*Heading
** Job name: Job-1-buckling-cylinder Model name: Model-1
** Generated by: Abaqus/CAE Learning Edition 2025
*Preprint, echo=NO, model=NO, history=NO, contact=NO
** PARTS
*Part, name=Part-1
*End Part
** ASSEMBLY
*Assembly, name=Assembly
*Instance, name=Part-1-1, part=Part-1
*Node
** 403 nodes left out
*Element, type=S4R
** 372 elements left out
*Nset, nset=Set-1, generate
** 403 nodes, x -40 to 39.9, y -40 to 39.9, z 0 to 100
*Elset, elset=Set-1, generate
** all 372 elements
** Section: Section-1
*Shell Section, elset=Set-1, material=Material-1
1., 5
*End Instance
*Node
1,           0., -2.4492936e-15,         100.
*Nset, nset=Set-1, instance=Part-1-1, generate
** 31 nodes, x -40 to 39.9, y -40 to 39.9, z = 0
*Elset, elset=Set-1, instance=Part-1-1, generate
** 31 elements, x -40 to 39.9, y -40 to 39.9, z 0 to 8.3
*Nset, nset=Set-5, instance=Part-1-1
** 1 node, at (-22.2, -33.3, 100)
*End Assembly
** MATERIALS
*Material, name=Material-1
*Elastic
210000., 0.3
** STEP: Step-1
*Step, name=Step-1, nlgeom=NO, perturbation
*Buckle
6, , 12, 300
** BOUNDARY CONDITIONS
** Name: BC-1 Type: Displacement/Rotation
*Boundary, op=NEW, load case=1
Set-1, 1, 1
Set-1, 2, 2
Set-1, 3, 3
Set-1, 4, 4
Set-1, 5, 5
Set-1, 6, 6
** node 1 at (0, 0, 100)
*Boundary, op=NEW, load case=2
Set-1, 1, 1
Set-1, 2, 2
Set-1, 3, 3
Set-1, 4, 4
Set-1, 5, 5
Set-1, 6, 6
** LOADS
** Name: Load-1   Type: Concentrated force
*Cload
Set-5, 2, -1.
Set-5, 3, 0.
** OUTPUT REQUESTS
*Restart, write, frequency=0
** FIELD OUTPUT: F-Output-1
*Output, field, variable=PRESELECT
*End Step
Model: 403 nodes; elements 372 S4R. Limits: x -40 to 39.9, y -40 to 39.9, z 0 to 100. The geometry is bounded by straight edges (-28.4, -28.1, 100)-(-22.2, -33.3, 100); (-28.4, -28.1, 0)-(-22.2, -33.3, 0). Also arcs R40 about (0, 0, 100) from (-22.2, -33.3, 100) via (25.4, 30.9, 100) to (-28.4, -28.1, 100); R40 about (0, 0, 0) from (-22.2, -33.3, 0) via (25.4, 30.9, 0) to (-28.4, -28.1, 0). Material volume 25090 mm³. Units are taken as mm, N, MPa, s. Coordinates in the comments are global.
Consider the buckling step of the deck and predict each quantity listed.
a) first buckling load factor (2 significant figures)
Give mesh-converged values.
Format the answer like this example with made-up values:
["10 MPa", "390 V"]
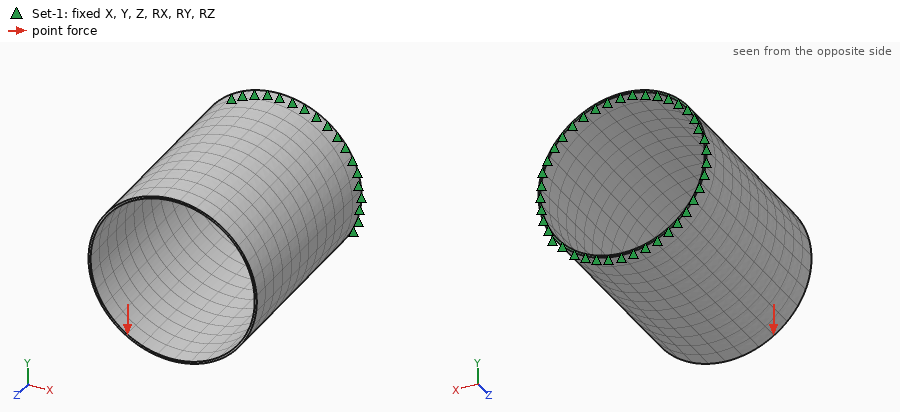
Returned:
["23000"]
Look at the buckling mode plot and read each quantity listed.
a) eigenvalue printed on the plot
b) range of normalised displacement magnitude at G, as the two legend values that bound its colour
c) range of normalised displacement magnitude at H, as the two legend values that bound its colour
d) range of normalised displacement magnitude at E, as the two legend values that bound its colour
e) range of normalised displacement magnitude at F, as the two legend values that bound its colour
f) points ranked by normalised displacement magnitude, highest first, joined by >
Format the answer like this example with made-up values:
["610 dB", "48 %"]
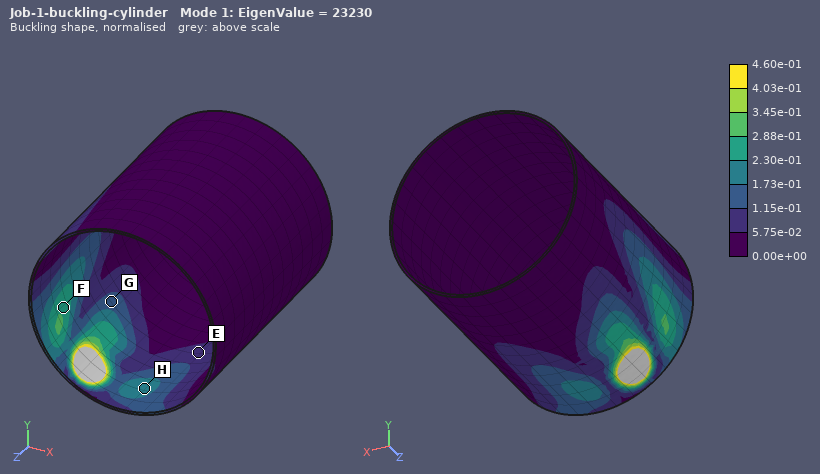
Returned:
["23230", "1.15e-01 to 1.73e-01", "1.73e-01 to 2.30e-01", "5.75e-02 to 1.15e-01", "2.30e-01 to 2.88e-01", "F > H > G > E"]
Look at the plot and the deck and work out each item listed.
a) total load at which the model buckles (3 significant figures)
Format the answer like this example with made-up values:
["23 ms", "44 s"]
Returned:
["23200 N"]
